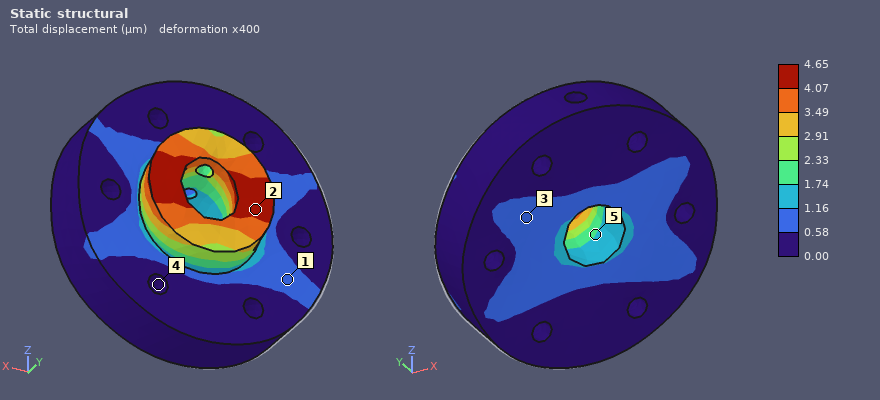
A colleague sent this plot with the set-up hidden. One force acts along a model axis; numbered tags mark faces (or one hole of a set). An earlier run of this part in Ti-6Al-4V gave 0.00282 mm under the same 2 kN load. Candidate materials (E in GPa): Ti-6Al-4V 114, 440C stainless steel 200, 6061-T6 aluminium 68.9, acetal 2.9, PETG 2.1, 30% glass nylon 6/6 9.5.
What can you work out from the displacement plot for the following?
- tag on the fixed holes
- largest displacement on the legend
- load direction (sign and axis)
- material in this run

4
4.65 µm
+X
6061-T6 aluminium
